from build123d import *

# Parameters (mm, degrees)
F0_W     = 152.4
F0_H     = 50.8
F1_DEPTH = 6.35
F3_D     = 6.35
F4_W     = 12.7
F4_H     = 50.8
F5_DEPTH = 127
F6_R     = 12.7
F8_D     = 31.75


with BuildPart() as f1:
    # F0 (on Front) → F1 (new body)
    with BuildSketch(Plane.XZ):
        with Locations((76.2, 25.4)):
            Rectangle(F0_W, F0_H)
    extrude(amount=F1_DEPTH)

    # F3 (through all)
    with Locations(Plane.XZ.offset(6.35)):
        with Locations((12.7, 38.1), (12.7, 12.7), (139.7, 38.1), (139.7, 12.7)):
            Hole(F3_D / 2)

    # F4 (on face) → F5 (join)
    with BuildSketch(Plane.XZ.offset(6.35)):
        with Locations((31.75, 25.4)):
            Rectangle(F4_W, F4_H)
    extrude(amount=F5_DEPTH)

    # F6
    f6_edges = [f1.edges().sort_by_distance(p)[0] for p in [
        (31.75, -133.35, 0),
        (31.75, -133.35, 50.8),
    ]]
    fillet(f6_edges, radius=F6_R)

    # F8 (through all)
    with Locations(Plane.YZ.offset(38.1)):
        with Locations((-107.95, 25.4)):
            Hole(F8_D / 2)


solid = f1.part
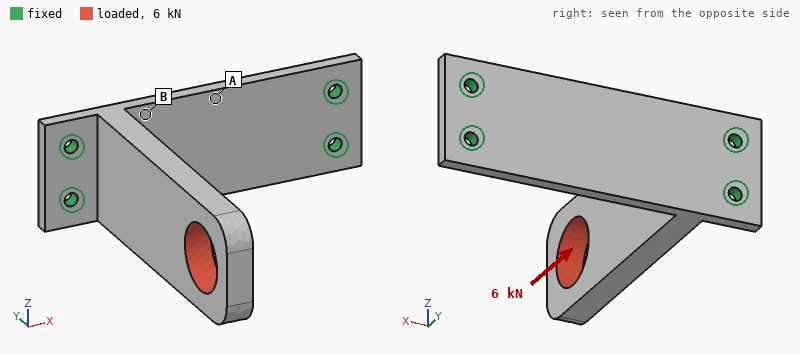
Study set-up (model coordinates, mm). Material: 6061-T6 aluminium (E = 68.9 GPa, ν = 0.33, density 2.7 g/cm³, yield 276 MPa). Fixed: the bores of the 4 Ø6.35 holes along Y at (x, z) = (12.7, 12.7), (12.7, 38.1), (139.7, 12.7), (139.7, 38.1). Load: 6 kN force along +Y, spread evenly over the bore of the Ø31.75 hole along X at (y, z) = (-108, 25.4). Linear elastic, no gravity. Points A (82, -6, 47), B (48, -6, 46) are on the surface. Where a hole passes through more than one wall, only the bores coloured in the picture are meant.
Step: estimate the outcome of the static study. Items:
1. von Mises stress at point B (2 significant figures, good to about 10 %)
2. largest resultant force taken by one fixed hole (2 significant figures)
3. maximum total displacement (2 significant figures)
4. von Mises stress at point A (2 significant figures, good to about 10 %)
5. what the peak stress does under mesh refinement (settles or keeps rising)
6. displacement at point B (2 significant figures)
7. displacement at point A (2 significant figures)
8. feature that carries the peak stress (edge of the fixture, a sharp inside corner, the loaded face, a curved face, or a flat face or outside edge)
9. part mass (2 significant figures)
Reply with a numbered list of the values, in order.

1. 59 MPa
2. 2.8 kN
3. 0.90 mm
4. 22 MPa
5. keeps rising
6. 0.20 mm
7. 0.17 mm
8. edge of the fixture
9. 320 g
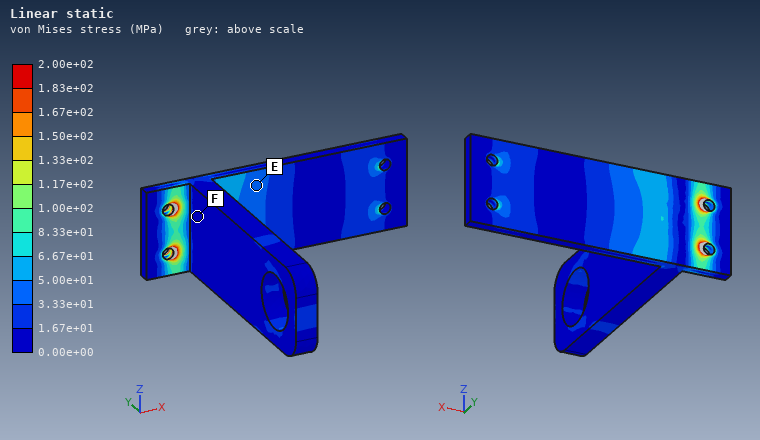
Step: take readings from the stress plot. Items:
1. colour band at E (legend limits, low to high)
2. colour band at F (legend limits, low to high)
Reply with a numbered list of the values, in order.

1. 3.33e+01 to 5.00e+01 MPa
2. 0.00e+00 to 1.67e+01 MPa
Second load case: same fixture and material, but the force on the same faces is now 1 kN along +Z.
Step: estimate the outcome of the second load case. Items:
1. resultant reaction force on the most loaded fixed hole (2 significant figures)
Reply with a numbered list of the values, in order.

1. 3.2 kN
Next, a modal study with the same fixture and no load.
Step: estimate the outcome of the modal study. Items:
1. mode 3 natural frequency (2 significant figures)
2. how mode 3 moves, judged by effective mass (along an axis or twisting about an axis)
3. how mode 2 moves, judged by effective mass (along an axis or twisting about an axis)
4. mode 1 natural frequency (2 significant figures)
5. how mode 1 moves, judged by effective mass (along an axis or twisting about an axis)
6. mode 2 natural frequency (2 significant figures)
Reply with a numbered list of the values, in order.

1. 2200 Hz
2. along Y
3. along Z
4. 420 Hz
5. along X
6. 870 Hz
